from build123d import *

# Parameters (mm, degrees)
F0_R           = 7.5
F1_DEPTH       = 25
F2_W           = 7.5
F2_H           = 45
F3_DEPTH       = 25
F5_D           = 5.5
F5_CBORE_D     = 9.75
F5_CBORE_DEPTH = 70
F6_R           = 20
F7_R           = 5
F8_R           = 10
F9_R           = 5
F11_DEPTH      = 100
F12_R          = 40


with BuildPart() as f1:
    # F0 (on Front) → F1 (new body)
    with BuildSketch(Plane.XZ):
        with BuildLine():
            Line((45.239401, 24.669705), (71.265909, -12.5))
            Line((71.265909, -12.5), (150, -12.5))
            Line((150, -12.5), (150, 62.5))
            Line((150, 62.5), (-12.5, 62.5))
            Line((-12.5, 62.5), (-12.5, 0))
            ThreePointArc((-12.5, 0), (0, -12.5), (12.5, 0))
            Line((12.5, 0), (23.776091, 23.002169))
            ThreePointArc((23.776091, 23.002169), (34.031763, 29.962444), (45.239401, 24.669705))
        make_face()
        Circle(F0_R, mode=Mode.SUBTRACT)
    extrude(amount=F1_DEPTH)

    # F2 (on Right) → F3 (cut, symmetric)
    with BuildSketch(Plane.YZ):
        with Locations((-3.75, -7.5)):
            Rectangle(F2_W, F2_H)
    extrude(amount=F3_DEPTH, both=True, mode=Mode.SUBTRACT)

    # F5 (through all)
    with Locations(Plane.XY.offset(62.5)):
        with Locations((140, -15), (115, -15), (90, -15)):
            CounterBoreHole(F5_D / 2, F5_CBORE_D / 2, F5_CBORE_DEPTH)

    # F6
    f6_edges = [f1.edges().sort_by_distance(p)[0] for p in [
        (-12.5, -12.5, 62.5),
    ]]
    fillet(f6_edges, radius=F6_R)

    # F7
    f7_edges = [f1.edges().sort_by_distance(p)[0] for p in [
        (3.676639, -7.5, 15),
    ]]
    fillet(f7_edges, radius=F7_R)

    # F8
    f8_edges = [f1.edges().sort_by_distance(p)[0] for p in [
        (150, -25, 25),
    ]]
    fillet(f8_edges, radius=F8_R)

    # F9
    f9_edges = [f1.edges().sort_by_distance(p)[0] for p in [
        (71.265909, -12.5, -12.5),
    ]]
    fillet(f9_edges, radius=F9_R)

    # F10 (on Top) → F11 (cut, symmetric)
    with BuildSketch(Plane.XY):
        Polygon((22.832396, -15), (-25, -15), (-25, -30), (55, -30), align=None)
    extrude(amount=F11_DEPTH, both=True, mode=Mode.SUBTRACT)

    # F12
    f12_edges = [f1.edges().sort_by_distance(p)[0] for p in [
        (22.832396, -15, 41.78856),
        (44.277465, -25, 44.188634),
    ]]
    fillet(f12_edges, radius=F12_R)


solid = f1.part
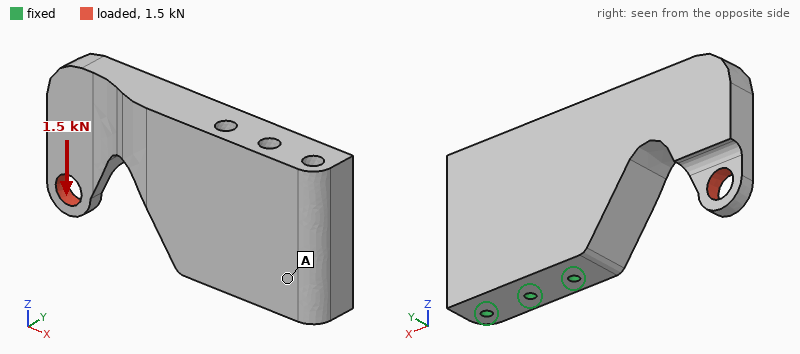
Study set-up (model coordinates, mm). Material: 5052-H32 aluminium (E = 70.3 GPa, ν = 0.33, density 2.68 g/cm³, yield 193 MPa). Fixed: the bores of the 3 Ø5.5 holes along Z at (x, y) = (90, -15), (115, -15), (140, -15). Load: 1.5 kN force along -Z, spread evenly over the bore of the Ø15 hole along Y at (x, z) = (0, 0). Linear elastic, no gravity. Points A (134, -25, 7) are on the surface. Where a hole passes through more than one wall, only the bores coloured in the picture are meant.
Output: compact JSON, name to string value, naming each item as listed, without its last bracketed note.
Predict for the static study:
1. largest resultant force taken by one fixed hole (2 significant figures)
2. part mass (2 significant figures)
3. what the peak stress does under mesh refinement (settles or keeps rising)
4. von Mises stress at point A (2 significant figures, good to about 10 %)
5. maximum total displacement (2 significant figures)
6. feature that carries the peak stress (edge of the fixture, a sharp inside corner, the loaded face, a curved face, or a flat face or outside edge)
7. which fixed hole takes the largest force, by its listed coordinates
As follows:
{"largest resultant force taken by one fixed hole": "4.0 kN", "part mass": "560 g", "what the peak stress does under mesh refinement": "keeps rising", "von Mises stress at point A": "8.5 MPa", "maximum total displacement": "0.10 mm", "feature that carries the peak stress": "edge of the fixture", "which fixed hole takes the largest force, by its listed coordinates": "(90, -15)"}
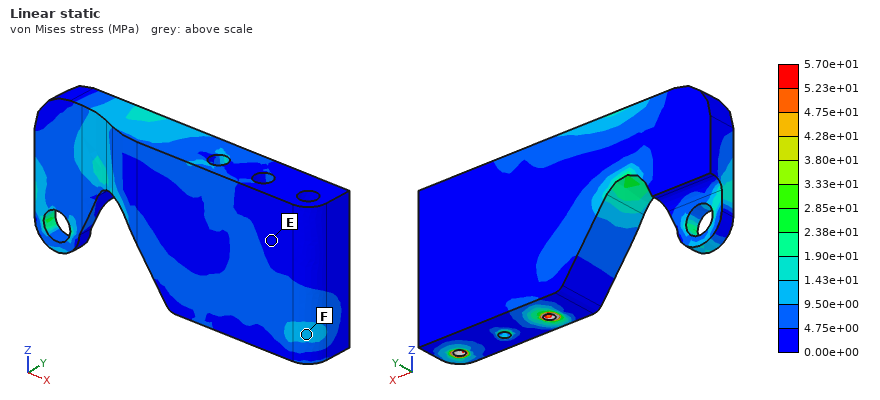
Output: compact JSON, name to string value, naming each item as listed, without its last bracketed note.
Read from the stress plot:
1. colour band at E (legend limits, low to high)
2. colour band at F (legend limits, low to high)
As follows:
{"colour band at E": "0.00e+00 to 4.75e+00 MPa", "colour band at F": "9.50e+00 to 1.43e+01 MPa"}
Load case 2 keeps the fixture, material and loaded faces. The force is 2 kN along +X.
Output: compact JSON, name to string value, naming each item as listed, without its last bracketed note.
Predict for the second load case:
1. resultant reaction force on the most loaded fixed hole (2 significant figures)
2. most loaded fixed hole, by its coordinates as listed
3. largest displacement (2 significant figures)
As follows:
{"resultant reaction force on the most loaded fixed hole": "1.1 kN", "most loaded fixed hole, by its coordinates as listed": "(90, -15)", "largest displacement": "0.11 mm"}
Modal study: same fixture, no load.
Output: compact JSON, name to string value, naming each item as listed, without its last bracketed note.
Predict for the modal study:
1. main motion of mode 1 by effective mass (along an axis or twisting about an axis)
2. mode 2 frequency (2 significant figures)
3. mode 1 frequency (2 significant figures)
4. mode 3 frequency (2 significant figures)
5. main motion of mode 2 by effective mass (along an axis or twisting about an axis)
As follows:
{"main motion of mode 1 by effective mass": "along Y", "mode 2 frequency": "1700 Hz", "mode 1 frequency": "740 Hz", "mode 3 frequency": "2000 Hz", "main motion of mode 2 by effective mass": "twisting about Z"}
